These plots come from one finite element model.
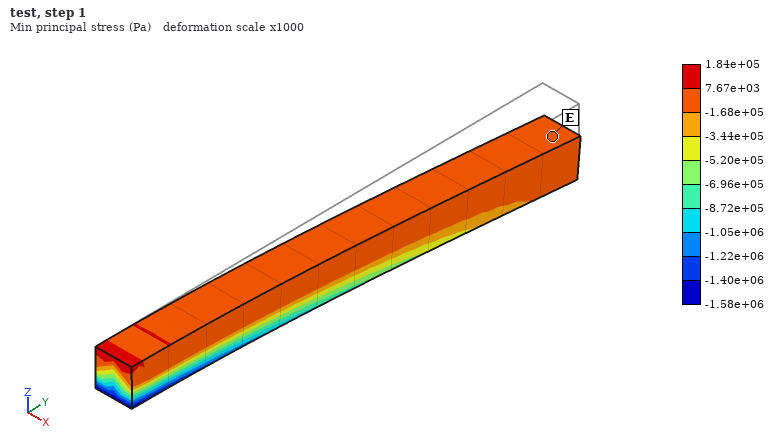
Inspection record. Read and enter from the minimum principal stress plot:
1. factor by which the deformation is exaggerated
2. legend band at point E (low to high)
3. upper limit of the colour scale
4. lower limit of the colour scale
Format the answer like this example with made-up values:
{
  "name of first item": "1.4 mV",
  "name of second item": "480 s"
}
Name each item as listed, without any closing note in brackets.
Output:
{
  "factor by which the deformation is exaggerated": "1000",
  "legend band at point E": "-1.68e+05 to 7.67e+03 Pa",
  "upper limit of the colour scale": "1.84e+05 Pa",
  "lower limit of the colour scale": "-1.58e+06 Pa"
}
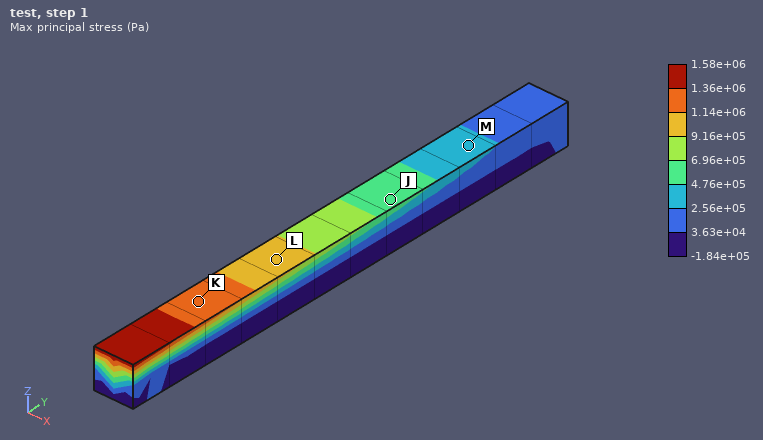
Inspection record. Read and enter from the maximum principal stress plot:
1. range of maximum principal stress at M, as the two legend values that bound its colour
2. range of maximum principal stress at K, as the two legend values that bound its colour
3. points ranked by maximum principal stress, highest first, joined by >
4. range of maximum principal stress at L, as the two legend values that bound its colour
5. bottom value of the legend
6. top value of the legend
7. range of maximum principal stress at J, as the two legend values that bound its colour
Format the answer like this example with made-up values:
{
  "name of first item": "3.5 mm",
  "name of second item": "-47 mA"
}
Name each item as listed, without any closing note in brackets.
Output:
{
  "range of maximum principal stress at M, as the two legend values that bound its colour": "2.56e+05 to 4.76e+05 Pa",
  "range of maximum principal stress at K, as the two legend values that bound its colour": "1.14e+06 to 1.36e+06 Pa",
  "points ranked by maximum principal stress, highest first, joined by >": "K > L > J > M",
  "range of maximum principal stress at L, as the two legend values that bound its colour": "9.16e+05 to 1.14e+06 Pa",
  "bottom value of the legend": "-1.84e+05 Pa",
  "top value of the legend": "1.58e+06 Pa",
  "range of maximum principal stress at J, as the two legend values that bound its colour": "4.76e+05 to 6.96e+05 Pa"
}
